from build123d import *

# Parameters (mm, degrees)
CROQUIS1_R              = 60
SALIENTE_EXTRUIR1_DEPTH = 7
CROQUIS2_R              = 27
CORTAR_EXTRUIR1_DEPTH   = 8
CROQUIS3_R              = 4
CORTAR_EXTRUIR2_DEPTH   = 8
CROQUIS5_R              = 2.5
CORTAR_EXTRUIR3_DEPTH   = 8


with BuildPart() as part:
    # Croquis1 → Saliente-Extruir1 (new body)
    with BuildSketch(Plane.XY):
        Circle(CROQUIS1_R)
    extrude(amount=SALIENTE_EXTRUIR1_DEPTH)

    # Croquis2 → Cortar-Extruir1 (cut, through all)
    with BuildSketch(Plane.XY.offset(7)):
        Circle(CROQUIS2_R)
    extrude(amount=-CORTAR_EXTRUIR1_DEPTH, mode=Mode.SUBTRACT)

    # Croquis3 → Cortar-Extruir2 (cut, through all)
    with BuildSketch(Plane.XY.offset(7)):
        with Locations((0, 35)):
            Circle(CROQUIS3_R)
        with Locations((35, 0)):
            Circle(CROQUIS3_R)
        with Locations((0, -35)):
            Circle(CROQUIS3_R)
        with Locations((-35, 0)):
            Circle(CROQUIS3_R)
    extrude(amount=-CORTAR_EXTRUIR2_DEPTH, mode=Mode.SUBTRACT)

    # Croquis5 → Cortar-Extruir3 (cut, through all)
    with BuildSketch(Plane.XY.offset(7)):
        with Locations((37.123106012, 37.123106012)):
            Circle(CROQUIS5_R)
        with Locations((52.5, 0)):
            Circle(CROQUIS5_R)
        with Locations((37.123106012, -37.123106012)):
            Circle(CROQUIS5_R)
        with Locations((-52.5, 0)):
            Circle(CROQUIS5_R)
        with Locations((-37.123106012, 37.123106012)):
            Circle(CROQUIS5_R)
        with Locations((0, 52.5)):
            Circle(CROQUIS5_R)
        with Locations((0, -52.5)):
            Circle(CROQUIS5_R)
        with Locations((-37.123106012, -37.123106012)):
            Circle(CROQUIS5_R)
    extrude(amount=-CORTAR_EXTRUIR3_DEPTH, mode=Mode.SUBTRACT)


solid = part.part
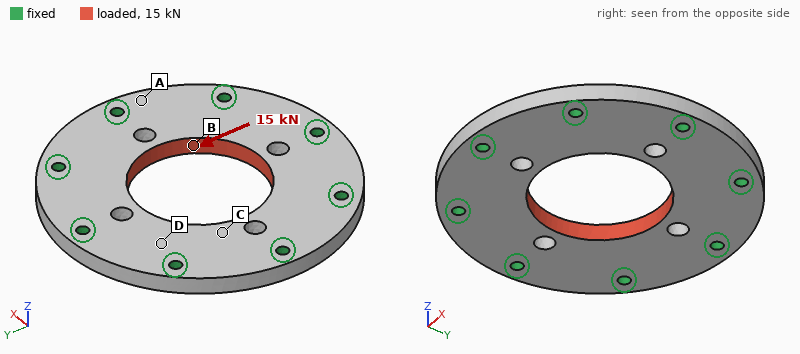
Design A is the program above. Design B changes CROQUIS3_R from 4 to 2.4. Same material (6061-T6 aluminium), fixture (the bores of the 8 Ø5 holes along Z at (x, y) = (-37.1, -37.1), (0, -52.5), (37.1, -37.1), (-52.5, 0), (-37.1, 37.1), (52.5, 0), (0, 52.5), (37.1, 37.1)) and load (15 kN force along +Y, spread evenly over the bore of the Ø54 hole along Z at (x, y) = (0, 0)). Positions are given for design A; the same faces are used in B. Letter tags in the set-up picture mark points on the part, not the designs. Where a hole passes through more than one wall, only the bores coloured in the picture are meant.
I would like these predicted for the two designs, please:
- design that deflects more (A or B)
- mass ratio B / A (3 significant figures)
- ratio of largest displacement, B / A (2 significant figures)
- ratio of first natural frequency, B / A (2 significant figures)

A
1.01
0.77
0.99
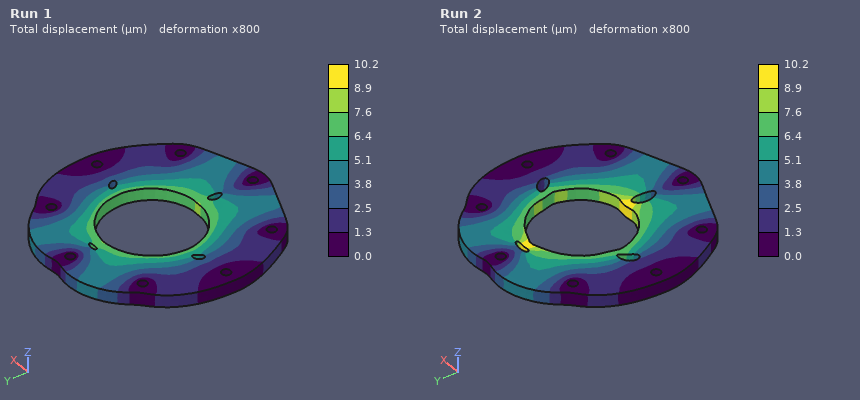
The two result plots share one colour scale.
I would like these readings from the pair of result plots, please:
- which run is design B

Run 1
